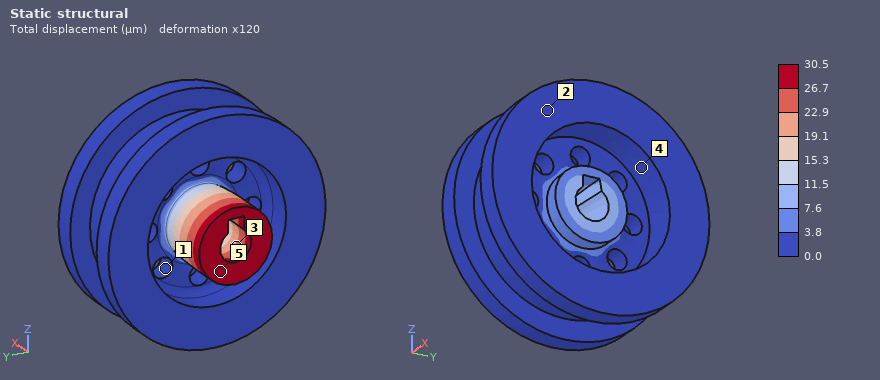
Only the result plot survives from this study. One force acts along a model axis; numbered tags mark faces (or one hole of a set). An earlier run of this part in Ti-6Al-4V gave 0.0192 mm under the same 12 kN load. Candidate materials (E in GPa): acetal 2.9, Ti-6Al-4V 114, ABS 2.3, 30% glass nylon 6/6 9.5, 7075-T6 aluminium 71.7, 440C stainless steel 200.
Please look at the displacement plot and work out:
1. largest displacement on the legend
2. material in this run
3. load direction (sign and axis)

30.5 µm
7075-T6 aluminium
+X
